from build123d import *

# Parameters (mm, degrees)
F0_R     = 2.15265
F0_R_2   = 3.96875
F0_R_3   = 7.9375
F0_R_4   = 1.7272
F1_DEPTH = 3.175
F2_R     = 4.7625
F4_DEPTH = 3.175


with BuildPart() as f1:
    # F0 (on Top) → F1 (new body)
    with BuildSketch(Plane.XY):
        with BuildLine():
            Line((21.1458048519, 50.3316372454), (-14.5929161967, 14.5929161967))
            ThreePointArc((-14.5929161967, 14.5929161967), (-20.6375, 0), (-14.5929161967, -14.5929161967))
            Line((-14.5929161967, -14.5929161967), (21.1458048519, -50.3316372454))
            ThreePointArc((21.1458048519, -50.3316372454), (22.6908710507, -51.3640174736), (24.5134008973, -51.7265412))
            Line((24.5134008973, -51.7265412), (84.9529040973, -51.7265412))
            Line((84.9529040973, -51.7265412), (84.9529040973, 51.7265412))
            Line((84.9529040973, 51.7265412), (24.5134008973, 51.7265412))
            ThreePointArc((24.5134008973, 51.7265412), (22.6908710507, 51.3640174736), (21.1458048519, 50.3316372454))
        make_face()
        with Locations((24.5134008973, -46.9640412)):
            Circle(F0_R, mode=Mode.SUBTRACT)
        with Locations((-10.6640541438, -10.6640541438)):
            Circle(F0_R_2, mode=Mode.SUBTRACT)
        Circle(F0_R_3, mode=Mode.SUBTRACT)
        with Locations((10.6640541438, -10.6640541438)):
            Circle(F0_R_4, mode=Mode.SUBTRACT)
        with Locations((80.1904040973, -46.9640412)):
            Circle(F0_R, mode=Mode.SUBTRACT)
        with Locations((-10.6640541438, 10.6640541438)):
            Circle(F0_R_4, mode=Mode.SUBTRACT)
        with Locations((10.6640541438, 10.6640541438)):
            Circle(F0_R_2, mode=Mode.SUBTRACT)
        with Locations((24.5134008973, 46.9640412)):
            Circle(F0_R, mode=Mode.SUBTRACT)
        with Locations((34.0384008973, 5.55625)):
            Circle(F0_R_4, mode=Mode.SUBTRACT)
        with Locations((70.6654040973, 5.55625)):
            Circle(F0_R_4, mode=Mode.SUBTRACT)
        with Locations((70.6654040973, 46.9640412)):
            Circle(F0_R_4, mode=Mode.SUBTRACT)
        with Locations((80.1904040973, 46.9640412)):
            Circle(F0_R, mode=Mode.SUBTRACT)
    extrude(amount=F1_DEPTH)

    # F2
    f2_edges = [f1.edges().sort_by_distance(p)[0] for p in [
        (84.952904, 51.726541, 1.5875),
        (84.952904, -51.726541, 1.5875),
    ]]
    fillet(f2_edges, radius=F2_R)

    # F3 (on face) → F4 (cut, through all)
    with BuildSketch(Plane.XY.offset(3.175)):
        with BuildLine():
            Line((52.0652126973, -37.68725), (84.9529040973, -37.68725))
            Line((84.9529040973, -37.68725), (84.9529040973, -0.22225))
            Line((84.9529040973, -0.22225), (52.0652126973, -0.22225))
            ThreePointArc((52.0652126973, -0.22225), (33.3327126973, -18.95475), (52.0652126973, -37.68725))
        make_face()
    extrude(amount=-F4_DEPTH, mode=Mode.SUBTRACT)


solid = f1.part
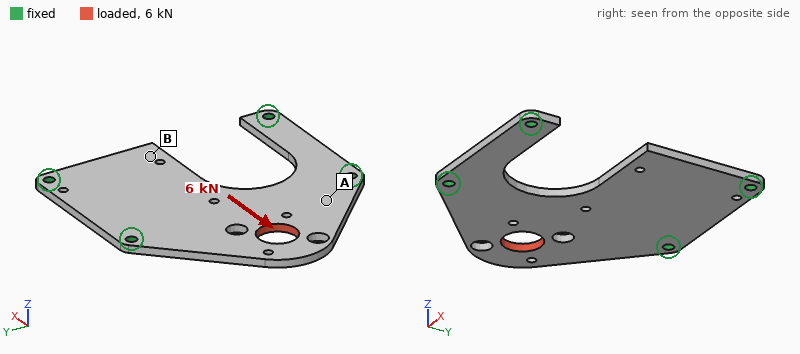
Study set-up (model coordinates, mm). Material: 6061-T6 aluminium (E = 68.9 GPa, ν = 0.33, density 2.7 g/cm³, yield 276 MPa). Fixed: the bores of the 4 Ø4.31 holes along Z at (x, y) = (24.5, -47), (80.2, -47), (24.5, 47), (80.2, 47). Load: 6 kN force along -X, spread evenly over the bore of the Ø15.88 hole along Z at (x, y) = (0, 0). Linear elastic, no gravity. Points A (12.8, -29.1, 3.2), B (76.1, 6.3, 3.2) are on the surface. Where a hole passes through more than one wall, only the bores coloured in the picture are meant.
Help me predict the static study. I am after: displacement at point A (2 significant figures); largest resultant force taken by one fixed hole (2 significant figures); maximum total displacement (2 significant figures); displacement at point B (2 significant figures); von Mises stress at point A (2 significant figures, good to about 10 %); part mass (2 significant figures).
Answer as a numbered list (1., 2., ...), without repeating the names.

1. 29 µm
2. 2.5 kN
3. 64 µm
4. 29 µm
5. 41 MPa
6. 59 g
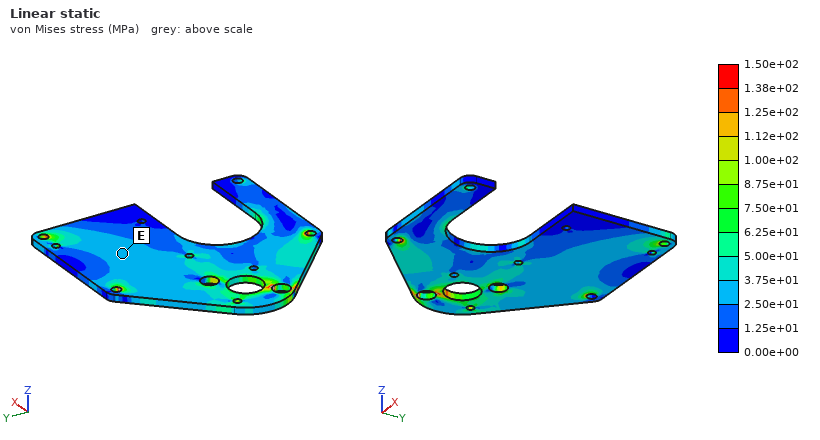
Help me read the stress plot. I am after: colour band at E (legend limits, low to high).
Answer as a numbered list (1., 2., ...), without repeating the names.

1. 2.50e+01 to 3.75e+01 MPa
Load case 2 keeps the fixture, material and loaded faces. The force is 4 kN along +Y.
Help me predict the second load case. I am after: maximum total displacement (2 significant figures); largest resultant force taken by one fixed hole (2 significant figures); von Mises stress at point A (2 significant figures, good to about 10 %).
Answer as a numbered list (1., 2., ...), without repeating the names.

1. 42 µm
2. 2.2 kN
3. 32 MPa
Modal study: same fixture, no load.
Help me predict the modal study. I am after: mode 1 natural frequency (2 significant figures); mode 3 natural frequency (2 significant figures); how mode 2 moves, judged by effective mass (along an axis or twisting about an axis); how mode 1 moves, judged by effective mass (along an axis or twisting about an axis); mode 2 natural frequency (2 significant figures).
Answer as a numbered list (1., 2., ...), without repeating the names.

1. 1100 Hz
2. 2800 Hz
3. along Z
4. along Z
5. 1400 Hz
